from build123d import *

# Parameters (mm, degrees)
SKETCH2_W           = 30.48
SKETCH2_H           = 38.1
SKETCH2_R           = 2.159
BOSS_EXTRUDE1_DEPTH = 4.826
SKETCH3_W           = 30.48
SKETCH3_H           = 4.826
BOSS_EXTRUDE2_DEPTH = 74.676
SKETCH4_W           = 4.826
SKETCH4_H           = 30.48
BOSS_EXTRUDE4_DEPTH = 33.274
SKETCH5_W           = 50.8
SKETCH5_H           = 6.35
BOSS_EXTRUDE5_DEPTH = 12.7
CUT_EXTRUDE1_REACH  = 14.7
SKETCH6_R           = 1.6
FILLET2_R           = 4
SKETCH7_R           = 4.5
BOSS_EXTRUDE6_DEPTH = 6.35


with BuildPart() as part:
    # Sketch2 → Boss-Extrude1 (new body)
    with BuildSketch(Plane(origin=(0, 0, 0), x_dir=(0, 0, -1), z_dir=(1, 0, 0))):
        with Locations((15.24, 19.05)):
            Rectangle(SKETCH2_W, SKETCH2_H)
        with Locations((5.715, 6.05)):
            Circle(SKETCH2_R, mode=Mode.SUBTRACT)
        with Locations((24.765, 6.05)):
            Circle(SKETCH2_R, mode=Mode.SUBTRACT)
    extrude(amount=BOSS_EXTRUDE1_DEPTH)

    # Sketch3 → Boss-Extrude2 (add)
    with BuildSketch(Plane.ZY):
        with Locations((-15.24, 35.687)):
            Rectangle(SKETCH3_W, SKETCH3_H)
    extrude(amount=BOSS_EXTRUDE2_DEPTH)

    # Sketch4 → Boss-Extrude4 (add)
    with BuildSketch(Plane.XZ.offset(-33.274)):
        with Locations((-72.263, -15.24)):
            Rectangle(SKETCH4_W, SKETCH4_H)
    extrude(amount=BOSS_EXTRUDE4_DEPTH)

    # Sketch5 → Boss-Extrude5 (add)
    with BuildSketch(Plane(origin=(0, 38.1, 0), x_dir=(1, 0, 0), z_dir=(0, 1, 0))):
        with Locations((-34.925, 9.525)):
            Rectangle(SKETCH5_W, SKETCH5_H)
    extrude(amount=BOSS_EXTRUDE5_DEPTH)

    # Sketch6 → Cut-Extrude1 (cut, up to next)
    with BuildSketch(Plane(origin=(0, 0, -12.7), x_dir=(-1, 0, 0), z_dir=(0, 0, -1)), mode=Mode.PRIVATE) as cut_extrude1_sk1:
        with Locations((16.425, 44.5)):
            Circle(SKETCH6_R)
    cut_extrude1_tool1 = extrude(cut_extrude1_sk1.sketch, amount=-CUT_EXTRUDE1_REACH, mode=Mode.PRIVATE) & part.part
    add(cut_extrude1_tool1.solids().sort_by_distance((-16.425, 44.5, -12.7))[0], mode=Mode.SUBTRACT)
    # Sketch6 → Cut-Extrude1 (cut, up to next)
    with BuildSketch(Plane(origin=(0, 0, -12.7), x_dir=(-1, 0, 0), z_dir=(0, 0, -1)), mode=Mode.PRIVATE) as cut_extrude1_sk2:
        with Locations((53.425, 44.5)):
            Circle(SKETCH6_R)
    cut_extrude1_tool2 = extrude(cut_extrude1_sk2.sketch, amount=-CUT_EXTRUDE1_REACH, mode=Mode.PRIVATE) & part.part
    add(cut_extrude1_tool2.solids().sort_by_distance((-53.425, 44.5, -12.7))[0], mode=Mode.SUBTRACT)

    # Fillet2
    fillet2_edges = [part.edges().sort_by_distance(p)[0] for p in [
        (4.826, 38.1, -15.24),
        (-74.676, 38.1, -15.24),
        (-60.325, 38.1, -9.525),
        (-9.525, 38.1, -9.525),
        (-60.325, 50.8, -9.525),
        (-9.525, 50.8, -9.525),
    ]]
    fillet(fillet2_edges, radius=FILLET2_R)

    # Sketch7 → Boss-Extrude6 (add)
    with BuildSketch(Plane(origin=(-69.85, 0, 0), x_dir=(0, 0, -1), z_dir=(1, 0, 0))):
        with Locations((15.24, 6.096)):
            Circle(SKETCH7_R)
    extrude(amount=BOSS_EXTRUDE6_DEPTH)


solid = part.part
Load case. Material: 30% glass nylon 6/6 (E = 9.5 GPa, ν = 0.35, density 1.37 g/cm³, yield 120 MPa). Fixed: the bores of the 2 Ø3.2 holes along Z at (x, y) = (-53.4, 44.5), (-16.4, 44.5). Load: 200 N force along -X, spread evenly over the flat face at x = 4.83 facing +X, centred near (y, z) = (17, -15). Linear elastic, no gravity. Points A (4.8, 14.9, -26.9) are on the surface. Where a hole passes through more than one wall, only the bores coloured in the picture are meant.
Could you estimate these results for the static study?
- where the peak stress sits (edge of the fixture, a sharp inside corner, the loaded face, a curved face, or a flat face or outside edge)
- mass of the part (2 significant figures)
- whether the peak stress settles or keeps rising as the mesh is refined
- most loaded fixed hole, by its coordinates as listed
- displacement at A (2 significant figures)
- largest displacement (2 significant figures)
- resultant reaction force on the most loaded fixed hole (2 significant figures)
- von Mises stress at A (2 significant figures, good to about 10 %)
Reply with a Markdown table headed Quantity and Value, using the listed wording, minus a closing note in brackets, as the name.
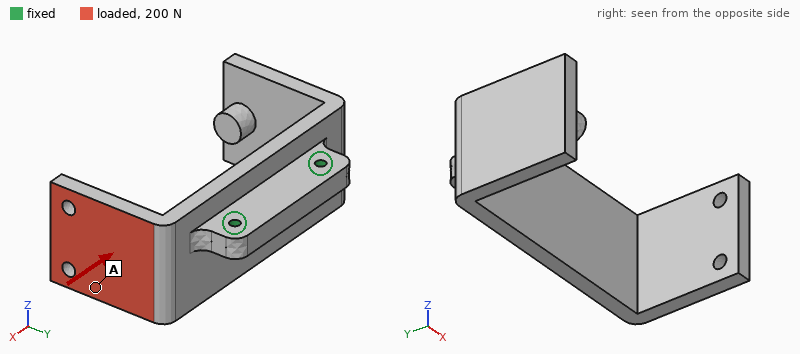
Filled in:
| Quantity | Value |
|---|---|
| where the peak stress sits | a sharp inside corner |
| mass of the part | 35 g |
| whether the peak stress settles or keeps rising as the mesh is refined | keeps rising |
| most loaded fixed hole, by its coordinates as listed | (-53.4, 44.5) |
| displacement at A | 0.67 mm |
| largest displacement | 1.2 mm |
| resultant reaction force on the most loaded fixed hole | 270 N |
| von Mises stress at A | 5.5 MPa |
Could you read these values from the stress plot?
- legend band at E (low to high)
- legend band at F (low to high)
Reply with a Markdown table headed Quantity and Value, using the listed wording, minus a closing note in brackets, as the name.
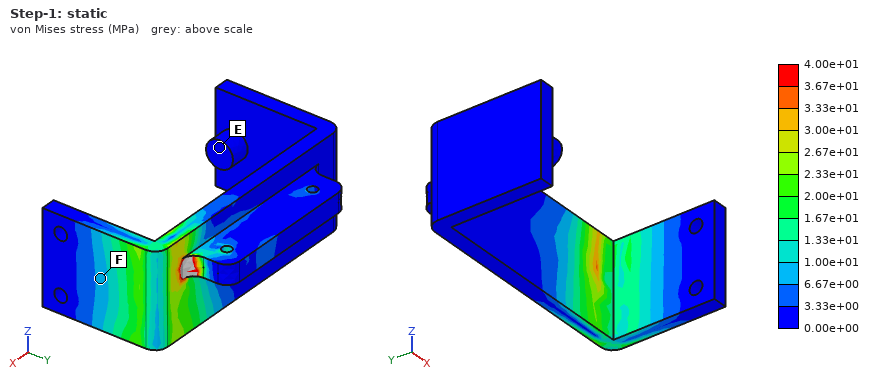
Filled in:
| Quantity | Value |
|---|---|
| legend band at E | 0.00e+00 to 3.33e+00 MPa |
| legend band at F | 6.67e+00 to 1.00e+01 MPa |
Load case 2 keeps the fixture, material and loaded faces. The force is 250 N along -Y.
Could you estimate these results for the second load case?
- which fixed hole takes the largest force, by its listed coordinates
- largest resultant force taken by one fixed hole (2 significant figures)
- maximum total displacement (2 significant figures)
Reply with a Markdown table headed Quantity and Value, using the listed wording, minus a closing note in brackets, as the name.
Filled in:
| Quantity | Value |
|---|---|
| which fixed hole takes the largest force, by its listed coordinates | (-16.4, 44.5) |
| largest resultant force taken by one fixed hole | 420 N |
| maximum total displacement | 0.81 mm |
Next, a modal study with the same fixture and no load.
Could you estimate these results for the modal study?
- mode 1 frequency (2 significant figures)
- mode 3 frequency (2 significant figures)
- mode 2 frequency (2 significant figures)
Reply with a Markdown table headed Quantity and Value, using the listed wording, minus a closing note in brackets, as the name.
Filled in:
| Quantity | Value |
|---|---|
| mode 1 frequency | 840 Hz |
| mode 3 frequency | 960 Hz |
| mode 2 frequency | 910 Hz |
